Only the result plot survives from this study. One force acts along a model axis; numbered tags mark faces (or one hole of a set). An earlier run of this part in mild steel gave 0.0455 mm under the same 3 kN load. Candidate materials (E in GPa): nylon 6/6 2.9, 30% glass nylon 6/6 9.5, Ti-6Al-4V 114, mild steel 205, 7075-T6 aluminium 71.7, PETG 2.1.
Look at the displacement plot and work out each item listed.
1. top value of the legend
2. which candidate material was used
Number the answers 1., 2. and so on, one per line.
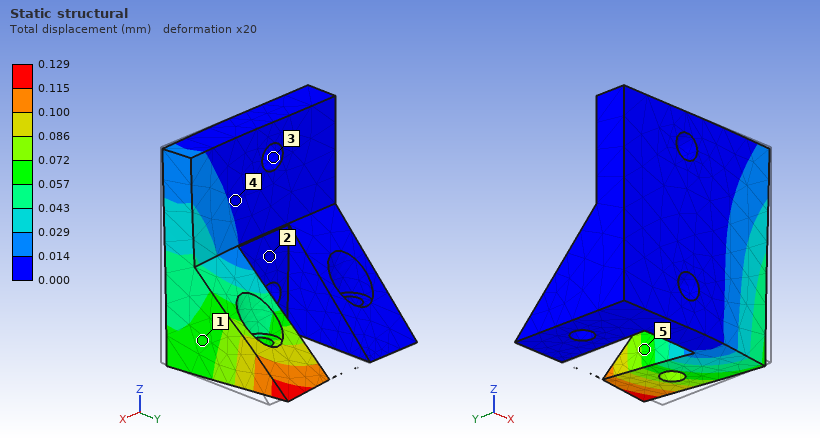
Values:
1. 0.129 mm
2. 7075-T6 aluminium
